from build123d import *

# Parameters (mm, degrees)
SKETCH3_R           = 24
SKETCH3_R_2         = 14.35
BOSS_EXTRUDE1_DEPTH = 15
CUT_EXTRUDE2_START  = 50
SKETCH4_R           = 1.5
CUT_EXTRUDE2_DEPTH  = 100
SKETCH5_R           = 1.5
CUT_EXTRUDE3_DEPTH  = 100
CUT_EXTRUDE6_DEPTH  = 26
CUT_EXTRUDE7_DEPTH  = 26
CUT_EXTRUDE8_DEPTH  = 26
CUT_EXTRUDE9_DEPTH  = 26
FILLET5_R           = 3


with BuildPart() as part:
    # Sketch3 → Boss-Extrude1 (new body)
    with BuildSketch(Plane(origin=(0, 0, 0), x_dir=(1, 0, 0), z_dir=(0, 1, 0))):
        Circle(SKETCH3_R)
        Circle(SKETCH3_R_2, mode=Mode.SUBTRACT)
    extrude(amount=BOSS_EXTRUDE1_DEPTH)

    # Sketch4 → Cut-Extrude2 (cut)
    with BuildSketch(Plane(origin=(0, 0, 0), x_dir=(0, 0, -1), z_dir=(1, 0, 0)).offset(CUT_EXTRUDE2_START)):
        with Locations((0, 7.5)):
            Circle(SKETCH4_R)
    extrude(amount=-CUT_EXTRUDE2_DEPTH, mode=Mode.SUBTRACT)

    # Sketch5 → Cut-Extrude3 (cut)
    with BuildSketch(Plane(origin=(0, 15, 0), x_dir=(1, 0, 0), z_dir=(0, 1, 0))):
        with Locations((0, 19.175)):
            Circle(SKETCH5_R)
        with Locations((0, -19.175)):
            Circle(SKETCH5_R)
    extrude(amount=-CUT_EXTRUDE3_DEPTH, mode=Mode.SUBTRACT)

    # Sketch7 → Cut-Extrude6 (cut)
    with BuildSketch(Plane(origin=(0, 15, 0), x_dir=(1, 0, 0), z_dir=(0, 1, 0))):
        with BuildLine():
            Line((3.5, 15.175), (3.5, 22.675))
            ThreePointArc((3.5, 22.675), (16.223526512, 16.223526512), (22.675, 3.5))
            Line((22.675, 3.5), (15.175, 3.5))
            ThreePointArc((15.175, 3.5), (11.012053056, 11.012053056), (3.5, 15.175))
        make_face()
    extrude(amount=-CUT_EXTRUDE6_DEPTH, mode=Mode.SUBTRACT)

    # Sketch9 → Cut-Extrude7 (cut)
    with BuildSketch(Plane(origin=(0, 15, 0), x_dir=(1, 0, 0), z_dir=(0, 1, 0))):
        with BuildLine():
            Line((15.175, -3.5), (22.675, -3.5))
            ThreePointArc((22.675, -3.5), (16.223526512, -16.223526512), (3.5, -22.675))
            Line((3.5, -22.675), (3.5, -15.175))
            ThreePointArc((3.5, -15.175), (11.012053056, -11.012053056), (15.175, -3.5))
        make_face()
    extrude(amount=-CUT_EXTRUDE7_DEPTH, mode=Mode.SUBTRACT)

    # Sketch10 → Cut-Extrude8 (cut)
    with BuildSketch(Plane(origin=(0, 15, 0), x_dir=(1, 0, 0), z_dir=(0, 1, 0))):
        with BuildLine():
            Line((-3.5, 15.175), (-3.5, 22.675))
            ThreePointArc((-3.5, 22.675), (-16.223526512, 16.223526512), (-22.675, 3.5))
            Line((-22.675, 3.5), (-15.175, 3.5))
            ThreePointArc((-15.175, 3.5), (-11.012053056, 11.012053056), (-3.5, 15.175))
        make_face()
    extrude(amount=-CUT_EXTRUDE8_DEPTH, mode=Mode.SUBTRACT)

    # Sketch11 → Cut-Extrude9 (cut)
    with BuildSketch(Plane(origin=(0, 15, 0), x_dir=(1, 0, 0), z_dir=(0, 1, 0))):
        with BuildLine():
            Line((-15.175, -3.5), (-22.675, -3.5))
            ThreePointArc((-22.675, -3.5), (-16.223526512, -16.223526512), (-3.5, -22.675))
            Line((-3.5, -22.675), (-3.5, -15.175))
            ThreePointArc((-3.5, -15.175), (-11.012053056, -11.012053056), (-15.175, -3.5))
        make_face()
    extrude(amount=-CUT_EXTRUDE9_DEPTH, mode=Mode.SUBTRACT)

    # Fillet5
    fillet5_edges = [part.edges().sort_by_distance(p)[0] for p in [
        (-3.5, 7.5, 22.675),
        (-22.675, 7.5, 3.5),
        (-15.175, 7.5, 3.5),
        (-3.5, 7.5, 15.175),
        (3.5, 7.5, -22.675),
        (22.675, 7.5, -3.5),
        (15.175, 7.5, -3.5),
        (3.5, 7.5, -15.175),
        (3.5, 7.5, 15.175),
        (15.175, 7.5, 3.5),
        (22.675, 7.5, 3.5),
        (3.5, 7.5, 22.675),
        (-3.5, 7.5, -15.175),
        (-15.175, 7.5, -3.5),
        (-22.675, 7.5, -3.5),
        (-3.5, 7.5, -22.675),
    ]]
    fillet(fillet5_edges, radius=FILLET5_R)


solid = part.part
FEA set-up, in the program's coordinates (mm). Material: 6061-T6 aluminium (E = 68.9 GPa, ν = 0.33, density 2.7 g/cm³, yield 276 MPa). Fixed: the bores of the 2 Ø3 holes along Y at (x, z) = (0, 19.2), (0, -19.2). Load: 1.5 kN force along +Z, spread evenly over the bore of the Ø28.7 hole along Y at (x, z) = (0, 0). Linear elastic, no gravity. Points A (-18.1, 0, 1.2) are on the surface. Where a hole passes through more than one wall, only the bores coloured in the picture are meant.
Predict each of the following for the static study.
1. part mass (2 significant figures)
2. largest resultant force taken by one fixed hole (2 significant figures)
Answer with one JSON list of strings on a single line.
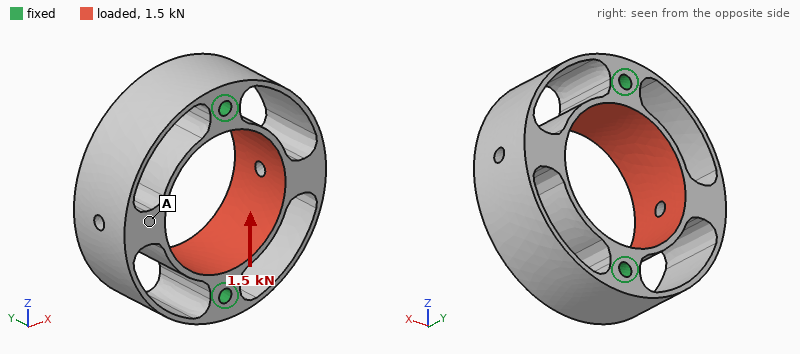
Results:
["20 g", "750 N"]
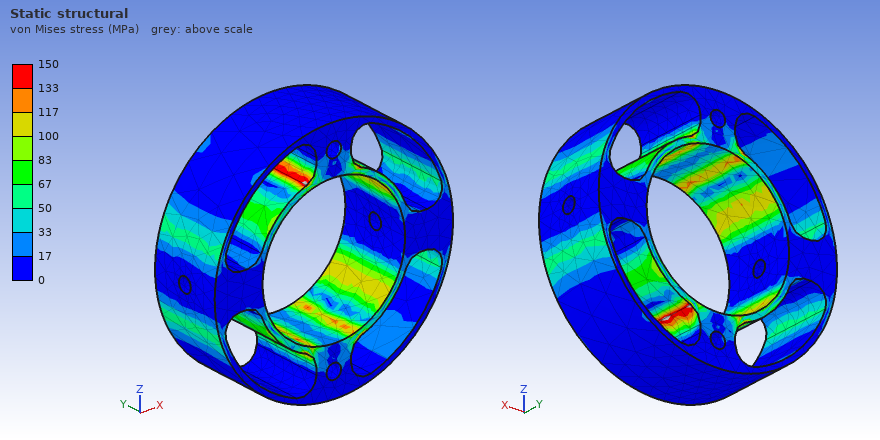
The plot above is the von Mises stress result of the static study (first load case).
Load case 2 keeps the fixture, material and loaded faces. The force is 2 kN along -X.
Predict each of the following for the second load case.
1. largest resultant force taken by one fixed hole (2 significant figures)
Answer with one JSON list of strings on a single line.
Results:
["1.0 kN"]
